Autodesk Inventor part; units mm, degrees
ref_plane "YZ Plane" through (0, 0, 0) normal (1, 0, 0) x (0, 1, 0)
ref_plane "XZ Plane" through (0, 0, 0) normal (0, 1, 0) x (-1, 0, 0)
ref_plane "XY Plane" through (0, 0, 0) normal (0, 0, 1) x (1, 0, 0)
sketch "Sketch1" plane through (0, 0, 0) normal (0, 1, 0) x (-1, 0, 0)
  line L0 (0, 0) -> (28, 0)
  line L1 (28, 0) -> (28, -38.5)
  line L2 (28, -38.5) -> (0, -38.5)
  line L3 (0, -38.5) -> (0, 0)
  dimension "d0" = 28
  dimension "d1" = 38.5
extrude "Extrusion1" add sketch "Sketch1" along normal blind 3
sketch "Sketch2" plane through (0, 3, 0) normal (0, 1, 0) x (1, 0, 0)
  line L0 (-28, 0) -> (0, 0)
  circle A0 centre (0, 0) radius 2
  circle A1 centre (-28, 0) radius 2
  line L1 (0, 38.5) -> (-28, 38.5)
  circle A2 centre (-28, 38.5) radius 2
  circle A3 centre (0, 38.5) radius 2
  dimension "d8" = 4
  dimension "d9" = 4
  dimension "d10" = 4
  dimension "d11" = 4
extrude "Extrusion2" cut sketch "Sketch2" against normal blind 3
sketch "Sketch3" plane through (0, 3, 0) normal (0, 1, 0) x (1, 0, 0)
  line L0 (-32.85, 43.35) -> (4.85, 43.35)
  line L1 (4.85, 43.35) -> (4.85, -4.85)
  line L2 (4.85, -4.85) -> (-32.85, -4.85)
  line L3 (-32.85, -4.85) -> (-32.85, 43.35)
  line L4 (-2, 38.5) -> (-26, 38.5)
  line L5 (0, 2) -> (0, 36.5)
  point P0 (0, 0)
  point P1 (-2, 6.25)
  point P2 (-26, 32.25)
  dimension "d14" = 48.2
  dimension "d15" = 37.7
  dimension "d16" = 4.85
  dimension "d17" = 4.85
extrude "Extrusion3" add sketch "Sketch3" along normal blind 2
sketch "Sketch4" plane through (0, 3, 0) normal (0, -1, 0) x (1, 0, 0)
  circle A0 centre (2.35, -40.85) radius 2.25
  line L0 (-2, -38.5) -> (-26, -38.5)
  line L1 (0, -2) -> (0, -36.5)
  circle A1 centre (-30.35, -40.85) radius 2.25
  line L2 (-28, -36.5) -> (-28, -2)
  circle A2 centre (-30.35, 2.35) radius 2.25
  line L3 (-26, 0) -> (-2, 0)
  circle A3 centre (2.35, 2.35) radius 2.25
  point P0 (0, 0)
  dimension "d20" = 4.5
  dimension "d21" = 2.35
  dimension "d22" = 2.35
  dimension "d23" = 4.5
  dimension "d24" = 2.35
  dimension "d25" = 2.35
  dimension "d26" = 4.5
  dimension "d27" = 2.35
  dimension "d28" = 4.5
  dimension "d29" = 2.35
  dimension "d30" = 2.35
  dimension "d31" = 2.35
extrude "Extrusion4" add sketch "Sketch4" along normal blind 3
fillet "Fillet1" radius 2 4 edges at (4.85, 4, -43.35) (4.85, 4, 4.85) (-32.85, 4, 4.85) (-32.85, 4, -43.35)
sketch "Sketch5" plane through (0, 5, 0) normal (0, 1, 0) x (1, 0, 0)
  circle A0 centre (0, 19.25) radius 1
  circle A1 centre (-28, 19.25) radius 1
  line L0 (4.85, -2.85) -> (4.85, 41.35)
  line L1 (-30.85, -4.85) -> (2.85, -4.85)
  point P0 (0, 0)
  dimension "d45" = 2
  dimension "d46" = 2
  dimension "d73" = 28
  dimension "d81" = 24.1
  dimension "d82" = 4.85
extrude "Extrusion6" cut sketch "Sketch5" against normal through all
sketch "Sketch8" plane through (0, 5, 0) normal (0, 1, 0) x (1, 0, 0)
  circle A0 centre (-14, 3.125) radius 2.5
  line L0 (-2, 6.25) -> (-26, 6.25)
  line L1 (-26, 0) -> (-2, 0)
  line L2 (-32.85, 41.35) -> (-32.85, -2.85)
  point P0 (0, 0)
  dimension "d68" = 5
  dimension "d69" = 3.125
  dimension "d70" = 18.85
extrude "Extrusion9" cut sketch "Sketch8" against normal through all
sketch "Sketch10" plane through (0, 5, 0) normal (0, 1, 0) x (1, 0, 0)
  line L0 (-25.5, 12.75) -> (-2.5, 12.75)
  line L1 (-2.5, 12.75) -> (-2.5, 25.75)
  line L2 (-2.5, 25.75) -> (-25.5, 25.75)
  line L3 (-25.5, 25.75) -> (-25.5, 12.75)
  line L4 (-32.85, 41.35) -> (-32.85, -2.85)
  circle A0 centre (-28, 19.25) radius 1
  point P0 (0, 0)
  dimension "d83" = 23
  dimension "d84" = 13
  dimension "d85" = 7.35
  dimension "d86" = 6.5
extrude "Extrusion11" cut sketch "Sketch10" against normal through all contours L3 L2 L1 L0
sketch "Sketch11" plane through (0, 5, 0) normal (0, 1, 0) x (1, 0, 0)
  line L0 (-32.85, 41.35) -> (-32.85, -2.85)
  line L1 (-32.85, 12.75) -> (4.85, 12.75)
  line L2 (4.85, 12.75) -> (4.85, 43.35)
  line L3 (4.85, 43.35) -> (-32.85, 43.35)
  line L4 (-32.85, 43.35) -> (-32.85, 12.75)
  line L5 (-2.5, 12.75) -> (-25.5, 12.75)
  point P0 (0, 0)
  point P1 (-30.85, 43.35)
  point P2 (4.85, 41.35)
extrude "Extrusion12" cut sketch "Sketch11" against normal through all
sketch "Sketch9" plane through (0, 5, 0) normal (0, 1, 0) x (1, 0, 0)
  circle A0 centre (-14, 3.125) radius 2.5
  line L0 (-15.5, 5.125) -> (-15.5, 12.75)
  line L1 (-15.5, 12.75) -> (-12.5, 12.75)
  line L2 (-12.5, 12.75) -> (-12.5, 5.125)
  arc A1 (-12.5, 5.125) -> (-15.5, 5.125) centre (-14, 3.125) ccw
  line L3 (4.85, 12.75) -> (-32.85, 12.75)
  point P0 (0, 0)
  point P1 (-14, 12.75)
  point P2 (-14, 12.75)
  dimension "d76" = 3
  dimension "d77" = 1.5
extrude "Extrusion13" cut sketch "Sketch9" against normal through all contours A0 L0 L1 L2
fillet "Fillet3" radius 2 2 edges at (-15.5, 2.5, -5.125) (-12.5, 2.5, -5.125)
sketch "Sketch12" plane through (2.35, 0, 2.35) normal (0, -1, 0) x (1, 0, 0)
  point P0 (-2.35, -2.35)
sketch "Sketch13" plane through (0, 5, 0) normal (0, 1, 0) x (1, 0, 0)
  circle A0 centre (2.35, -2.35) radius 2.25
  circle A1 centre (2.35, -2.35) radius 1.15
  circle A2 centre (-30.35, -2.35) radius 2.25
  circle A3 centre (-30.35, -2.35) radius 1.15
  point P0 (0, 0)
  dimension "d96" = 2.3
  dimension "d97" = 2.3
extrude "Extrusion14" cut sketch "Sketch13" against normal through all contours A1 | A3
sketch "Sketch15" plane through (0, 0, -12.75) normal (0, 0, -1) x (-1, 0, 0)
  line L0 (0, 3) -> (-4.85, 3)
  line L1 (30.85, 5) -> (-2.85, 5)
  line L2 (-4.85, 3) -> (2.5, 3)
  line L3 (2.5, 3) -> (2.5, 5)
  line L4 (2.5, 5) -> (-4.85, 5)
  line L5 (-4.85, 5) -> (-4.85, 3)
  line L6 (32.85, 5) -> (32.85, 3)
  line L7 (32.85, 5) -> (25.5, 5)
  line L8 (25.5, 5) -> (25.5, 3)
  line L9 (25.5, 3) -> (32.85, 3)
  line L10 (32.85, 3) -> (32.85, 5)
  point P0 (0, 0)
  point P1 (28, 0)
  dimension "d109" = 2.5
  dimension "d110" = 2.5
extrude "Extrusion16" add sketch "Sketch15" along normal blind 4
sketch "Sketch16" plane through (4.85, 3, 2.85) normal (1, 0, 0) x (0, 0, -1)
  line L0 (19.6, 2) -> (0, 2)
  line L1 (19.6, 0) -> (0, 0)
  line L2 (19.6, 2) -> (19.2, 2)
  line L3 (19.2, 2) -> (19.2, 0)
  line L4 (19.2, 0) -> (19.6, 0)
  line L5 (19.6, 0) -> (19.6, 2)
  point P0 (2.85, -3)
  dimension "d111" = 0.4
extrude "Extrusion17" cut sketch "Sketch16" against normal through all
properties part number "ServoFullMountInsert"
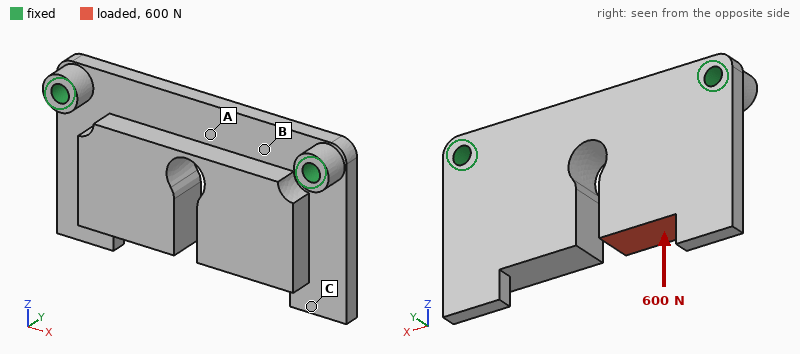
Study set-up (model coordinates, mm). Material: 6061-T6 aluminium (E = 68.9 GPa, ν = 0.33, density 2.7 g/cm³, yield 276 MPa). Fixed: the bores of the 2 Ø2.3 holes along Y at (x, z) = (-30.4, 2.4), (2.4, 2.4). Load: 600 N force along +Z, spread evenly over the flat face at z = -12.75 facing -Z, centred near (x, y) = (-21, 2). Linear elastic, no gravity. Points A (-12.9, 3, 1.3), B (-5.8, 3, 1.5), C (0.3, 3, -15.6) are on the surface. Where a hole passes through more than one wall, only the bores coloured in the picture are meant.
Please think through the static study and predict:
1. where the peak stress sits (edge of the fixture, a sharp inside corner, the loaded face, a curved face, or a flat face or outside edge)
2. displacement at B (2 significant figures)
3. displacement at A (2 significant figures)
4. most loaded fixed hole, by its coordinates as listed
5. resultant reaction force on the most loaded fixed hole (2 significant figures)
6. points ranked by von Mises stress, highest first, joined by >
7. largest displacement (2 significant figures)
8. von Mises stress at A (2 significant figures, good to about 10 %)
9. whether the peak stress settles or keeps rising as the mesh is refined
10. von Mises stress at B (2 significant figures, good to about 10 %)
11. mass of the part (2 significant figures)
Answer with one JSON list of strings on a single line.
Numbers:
["a sharp inside corner", "0.018 mm", "0.036 mm", "(-30.4, 2.4)", "460 N", "A > B > C", "0.12 mm", "78 MPa", "keeps rising", "38 MPa", "6.3 g"]
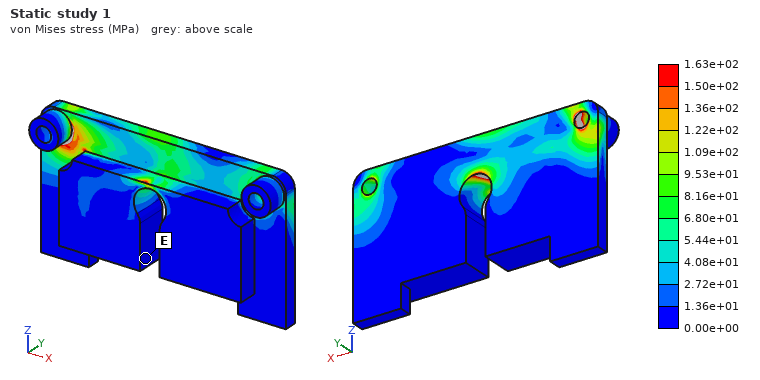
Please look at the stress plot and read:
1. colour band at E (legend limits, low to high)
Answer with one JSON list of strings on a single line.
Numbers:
["0.00e+00 to 1.36e+01 MPa"]
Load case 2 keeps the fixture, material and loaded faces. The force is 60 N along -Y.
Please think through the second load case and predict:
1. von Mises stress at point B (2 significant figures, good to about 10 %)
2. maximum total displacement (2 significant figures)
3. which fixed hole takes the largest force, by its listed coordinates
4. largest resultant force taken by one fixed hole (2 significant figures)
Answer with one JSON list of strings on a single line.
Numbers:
["12 MPa", "93 µm", "(-30.4, 2.4)", "50 N"]
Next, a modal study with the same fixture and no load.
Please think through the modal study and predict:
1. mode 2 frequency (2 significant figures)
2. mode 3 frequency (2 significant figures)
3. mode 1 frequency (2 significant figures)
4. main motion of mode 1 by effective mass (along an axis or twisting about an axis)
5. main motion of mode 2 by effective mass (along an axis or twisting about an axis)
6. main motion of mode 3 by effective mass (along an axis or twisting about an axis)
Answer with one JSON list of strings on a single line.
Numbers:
["5300 Hz", "8500 Hz", "3700 Hz", "along Y", "twisting about Z", "along Z"]
